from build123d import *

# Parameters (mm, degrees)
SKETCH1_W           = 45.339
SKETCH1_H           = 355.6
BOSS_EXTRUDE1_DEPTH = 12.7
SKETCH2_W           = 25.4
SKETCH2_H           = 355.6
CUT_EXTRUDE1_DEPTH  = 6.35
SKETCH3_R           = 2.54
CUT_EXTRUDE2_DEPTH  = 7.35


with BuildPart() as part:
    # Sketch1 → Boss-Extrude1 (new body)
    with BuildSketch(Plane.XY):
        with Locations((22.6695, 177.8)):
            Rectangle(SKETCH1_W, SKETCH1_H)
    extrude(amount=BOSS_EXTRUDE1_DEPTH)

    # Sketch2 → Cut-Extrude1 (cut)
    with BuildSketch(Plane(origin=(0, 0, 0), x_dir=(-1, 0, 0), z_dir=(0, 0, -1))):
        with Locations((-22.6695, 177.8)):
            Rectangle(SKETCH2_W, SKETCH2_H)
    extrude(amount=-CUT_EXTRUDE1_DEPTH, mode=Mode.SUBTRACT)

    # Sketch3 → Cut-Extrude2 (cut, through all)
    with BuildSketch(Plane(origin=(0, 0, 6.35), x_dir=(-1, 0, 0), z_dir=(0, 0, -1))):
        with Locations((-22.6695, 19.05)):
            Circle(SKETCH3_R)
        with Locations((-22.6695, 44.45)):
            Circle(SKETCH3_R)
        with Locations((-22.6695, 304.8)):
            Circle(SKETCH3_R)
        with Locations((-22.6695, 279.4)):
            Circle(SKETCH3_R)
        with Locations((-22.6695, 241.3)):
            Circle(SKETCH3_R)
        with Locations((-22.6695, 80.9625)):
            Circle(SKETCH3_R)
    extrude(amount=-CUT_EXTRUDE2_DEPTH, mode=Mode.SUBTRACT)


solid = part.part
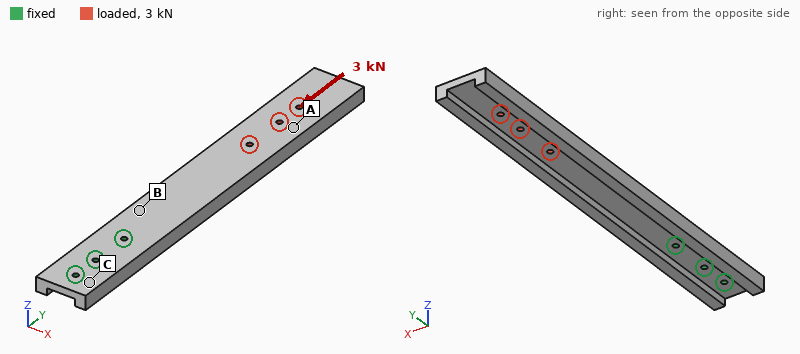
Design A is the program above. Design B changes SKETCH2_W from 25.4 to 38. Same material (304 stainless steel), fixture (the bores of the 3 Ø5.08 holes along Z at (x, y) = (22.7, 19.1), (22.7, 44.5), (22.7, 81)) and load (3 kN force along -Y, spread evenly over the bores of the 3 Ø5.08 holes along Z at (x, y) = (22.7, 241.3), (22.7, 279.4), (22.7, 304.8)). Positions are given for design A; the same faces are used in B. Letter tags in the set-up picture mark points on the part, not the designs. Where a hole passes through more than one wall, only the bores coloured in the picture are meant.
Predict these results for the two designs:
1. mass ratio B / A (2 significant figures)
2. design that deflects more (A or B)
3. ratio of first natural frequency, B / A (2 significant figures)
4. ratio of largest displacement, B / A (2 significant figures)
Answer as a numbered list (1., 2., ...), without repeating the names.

1. 0.81
2. A
3. 0.84
4. 0.80
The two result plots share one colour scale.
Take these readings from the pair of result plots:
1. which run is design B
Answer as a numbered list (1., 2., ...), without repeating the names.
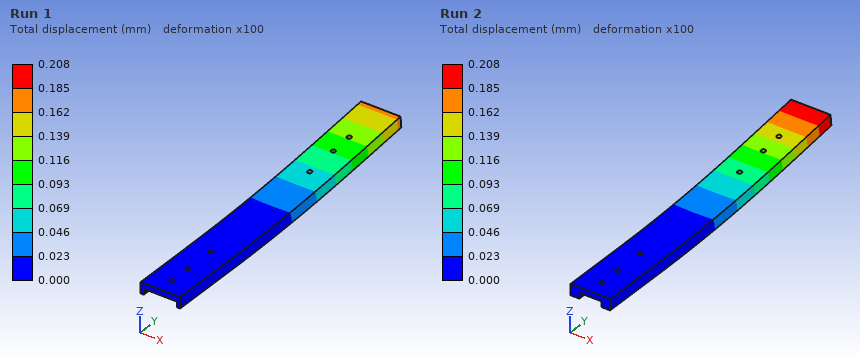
1. Run 1
